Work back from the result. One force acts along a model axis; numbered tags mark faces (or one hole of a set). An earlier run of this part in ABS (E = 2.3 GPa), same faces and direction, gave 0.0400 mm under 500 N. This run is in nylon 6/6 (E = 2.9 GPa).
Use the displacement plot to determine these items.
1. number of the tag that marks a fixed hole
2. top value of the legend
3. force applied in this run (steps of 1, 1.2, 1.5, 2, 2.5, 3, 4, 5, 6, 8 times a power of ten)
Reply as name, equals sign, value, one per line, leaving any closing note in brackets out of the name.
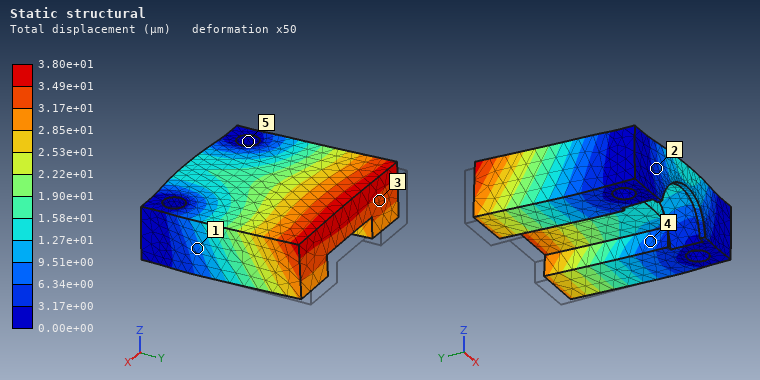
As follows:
number of the tag that marks a fixed hole = 5
top value of the legend = 3.80e+01 µm
force applied in this run = 600 N
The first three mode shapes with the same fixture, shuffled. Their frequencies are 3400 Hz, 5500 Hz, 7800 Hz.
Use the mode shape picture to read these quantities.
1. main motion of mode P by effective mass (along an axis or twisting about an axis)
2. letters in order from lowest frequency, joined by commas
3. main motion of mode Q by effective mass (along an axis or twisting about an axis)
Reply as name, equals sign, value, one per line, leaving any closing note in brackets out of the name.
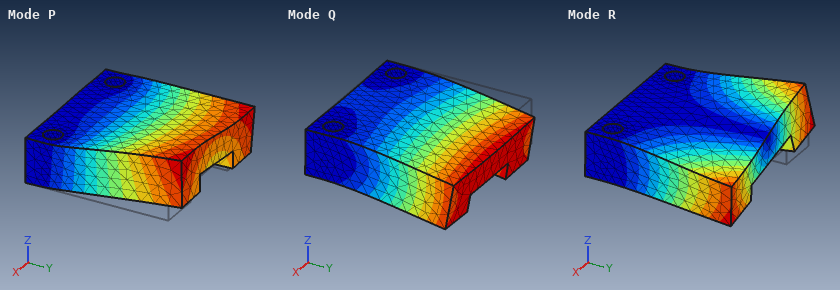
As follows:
main motion of mode P by effective mass = along X
letters in order from lowest frequency, joined by commas = Q, R, P
main motion of mode Q by effective mass = along Z
